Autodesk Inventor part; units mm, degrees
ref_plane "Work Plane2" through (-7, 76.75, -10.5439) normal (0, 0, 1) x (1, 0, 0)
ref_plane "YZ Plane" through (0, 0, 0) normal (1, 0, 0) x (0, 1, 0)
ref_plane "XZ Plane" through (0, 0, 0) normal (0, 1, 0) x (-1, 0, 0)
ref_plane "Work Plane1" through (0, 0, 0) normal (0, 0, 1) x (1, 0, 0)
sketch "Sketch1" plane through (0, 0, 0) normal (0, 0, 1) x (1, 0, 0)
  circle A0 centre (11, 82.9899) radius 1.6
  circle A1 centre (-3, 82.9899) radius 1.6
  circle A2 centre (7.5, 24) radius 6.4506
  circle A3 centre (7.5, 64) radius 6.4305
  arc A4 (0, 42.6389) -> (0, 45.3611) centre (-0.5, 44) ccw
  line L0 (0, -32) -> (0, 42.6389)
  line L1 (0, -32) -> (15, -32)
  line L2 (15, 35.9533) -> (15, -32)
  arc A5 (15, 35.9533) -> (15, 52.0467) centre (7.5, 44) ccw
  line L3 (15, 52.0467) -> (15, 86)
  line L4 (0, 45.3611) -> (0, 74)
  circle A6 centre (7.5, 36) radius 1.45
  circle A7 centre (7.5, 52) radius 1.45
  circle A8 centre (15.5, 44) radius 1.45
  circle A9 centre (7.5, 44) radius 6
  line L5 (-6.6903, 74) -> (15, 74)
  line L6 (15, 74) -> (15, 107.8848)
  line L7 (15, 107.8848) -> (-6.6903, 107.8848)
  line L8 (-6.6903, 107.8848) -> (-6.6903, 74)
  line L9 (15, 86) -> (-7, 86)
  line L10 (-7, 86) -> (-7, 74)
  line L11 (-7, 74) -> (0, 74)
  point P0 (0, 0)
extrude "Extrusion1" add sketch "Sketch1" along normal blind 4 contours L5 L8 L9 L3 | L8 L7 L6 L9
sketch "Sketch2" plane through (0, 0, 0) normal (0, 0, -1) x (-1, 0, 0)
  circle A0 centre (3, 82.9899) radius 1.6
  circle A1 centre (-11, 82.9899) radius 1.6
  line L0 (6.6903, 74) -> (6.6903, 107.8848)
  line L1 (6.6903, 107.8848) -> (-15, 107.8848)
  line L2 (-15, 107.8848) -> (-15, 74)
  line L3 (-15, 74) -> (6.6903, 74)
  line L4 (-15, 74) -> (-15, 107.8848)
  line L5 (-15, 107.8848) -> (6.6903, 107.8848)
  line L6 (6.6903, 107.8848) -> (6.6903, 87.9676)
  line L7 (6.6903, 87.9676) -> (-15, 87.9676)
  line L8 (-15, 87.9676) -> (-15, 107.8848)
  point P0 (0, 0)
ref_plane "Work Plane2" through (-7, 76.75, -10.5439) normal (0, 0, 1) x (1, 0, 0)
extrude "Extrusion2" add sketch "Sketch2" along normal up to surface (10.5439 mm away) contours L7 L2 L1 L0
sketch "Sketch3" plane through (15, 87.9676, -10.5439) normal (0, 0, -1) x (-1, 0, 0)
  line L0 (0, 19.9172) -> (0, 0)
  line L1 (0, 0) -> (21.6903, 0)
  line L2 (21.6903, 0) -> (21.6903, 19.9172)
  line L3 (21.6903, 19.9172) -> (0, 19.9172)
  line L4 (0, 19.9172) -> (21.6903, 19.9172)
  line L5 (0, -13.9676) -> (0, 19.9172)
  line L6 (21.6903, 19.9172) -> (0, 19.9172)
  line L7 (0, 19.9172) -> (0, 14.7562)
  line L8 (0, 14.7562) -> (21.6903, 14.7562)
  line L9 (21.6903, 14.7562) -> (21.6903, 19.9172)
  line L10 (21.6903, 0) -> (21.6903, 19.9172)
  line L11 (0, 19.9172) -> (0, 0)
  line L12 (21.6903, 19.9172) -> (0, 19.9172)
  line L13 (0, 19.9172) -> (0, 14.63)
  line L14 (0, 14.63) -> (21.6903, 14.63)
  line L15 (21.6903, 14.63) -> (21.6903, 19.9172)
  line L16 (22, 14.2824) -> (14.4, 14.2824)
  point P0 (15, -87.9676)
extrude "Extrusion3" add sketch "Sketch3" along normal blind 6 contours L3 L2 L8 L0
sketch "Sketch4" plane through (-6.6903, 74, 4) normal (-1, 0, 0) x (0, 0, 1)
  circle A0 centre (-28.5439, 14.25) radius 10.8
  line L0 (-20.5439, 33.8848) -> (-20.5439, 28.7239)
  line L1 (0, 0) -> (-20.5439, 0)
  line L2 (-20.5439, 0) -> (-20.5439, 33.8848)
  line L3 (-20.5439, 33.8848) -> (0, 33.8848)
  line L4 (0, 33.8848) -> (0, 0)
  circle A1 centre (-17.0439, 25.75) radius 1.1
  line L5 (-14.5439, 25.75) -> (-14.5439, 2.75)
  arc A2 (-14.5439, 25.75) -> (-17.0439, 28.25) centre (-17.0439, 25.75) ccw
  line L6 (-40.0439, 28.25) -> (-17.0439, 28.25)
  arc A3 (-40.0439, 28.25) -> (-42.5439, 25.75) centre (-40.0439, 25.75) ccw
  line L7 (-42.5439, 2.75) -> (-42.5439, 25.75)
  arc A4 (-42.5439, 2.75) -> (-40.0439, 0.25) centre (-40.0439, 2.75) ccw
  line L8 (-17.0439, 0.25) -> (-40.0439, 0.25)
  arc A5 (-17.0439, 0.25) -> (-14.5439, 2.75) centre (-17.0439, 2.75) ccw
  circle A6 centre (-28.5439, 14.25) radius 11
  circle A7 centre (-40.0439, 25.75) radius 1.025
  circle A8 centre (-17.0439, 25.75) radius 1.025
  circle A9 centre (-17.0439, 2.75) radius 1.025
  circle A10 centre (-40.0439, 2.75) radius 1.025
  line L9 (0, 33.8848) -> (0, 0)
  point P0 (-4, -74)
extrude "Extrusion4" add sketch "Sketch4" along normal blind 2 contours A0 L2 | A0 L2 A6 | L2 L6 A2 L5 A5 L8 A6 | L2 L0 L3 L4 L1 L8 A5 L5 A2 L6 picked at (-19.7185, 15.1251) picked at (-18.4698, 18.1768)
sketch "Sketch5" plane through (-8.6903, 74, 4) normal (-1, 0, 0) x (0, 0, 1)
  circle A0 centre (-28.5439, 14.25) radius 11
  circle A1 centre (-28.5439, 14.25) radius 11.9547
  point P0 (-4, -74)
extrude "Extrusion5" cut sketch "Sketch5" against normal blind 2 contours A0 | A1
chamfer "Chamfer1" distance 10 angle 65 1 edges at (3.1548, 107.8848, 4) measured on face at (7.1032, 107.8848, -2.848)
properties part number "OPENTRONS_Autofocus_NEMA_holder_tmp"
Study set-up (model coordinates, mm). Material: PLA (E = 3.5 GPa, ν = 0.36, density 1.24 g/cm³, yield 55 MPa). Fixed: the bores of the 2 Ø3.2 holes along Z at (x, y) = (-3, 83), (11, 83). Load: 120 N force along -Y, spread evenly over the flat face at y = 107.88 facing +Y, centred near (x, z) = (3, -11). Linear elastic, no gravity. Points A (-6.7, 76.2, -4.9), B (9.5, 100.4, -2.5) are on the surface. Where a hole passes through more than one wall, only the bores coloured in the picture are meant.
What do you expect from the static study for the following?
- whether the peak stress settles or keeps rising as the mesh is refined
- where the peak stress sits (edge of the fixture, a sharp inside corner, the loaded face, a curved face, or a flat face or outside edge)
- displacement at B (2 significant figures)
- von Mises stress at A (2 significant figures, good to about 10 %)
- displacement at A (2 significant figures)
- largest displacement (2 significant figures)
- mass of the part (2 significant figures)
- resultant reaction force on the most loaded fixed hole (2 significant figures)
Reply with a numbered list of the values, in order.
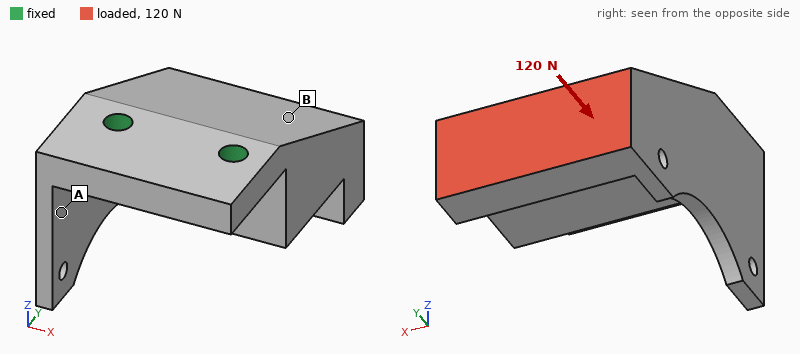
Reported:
1. keeps rising
2. edge of the fixture
3. 0.24 mm
4. 6.1 MPa
5. 0.13 mm
6. 0.50 mm
7. 8.5 g
8. 63 N
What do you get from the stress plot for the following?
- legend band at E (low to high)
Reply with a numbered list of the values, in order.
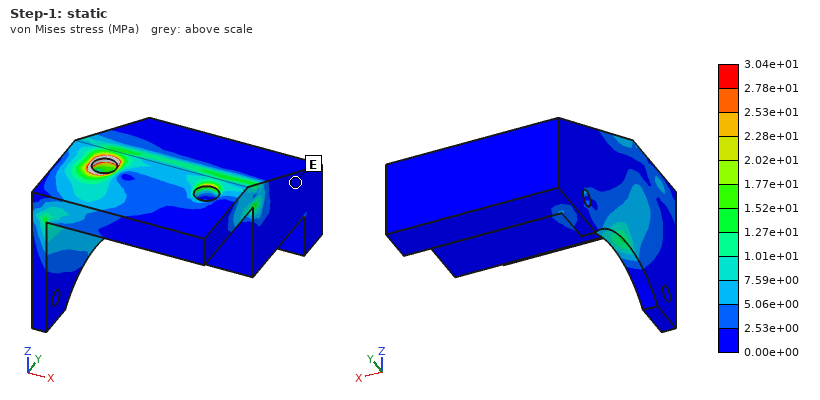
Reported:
1. 0.00e+00 to 2.53e+00 MPa
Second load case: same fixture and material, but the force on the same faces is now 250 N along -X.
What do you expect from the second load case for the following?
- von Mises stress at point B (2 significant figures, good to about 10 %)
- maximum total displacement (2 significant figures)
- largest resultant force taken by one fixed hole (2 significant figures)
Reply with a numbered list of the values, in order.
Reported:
1. 3.6 MPa
2. 0.29 mm
3. 460 N
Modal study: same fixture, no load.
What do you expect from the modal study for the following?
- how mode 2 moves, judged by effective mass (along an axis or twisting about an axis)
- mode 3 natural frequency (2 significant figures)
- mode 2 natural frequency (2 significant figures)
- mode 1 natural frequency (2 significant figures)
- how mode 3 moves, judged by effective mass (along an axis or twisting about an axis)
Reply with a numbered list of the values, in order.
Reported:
1. along X
2. 3500 Hz
3. 3000 Hz
4. 1200 Hz
5. along X
